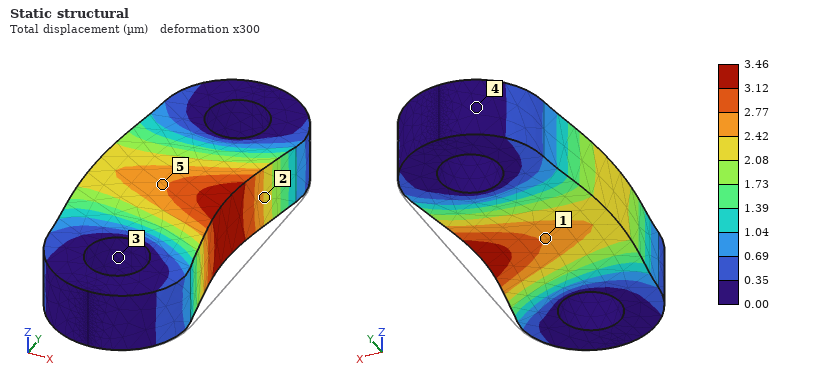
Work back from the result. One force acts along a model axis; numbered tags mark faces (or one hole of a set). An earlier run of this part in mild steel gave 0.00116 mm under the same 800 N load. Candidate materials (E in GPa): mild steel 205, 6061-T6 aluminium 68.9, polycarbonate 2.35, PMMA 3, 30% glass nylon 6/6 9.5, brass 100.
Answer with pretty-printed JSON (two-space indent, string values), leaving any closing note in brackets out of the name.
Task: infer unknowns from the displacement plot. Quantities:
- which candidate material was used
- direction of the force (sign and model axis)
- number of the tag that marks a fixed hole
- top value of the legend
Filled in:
{
  "which candidate material was used": "6061-T6 aluminium",
  "direction of the force": "-X",
  "number of the tag that marks a fixed hole": "3",
  "top value of the legend": "3.46 µm"
}
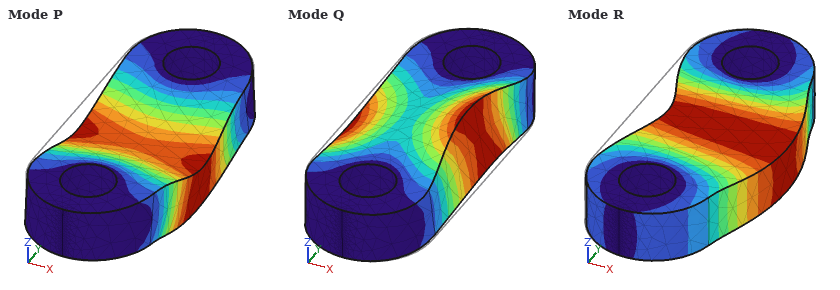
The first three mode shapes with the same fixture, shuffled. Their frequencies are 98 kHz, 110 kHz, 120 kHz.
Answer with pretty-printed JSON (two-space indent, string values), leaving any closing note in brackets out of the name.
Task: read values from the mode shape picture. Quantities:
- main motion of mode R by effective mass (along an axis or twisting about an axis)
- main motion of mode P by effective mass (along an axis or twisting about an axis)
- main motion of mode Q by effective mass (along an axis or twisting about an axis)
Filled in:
{
  "main motion of mode R by effective mass": "along X",
  "main motion of mode P by effective mass": "along Z",
  "main motion of mode Q by effective mass": "twisting about Y"
}
